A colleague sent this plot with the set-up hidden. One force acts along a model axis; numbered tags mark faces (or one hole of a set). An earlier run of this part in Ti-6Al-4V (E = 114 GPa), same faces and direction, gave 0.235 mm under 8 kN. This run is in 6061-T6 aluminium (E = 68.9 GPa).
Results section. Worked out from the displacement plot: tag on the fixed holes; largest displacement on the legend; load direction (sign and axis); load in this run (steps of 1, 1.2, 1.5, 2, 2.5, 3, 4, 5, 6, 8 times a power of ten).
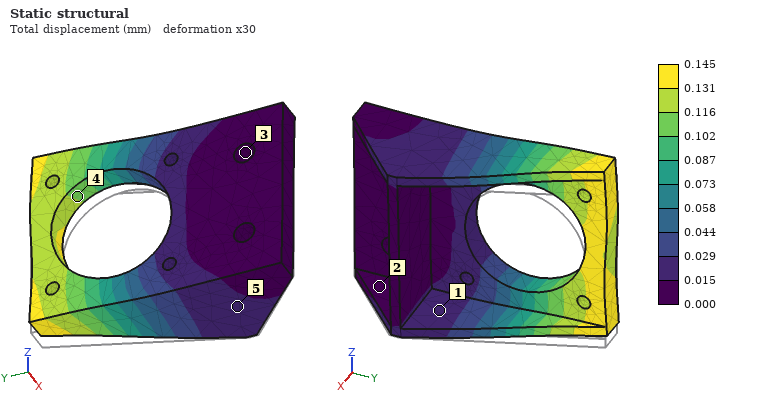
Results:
3
0.145 mm
+Z
3 kN
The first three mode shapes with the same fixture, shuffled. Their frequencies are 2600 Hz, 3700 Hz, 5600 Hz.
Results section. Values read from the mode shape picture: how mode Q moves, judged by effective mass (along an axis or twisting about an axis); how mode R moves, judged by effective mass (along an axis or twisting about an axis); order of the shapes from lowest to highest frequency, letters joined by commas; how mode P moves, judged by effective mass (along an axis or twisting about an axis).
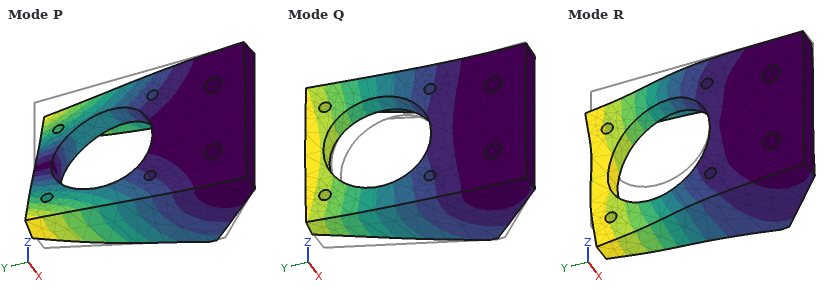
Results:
along X
along Z
Q, P, R
twisting about Y
